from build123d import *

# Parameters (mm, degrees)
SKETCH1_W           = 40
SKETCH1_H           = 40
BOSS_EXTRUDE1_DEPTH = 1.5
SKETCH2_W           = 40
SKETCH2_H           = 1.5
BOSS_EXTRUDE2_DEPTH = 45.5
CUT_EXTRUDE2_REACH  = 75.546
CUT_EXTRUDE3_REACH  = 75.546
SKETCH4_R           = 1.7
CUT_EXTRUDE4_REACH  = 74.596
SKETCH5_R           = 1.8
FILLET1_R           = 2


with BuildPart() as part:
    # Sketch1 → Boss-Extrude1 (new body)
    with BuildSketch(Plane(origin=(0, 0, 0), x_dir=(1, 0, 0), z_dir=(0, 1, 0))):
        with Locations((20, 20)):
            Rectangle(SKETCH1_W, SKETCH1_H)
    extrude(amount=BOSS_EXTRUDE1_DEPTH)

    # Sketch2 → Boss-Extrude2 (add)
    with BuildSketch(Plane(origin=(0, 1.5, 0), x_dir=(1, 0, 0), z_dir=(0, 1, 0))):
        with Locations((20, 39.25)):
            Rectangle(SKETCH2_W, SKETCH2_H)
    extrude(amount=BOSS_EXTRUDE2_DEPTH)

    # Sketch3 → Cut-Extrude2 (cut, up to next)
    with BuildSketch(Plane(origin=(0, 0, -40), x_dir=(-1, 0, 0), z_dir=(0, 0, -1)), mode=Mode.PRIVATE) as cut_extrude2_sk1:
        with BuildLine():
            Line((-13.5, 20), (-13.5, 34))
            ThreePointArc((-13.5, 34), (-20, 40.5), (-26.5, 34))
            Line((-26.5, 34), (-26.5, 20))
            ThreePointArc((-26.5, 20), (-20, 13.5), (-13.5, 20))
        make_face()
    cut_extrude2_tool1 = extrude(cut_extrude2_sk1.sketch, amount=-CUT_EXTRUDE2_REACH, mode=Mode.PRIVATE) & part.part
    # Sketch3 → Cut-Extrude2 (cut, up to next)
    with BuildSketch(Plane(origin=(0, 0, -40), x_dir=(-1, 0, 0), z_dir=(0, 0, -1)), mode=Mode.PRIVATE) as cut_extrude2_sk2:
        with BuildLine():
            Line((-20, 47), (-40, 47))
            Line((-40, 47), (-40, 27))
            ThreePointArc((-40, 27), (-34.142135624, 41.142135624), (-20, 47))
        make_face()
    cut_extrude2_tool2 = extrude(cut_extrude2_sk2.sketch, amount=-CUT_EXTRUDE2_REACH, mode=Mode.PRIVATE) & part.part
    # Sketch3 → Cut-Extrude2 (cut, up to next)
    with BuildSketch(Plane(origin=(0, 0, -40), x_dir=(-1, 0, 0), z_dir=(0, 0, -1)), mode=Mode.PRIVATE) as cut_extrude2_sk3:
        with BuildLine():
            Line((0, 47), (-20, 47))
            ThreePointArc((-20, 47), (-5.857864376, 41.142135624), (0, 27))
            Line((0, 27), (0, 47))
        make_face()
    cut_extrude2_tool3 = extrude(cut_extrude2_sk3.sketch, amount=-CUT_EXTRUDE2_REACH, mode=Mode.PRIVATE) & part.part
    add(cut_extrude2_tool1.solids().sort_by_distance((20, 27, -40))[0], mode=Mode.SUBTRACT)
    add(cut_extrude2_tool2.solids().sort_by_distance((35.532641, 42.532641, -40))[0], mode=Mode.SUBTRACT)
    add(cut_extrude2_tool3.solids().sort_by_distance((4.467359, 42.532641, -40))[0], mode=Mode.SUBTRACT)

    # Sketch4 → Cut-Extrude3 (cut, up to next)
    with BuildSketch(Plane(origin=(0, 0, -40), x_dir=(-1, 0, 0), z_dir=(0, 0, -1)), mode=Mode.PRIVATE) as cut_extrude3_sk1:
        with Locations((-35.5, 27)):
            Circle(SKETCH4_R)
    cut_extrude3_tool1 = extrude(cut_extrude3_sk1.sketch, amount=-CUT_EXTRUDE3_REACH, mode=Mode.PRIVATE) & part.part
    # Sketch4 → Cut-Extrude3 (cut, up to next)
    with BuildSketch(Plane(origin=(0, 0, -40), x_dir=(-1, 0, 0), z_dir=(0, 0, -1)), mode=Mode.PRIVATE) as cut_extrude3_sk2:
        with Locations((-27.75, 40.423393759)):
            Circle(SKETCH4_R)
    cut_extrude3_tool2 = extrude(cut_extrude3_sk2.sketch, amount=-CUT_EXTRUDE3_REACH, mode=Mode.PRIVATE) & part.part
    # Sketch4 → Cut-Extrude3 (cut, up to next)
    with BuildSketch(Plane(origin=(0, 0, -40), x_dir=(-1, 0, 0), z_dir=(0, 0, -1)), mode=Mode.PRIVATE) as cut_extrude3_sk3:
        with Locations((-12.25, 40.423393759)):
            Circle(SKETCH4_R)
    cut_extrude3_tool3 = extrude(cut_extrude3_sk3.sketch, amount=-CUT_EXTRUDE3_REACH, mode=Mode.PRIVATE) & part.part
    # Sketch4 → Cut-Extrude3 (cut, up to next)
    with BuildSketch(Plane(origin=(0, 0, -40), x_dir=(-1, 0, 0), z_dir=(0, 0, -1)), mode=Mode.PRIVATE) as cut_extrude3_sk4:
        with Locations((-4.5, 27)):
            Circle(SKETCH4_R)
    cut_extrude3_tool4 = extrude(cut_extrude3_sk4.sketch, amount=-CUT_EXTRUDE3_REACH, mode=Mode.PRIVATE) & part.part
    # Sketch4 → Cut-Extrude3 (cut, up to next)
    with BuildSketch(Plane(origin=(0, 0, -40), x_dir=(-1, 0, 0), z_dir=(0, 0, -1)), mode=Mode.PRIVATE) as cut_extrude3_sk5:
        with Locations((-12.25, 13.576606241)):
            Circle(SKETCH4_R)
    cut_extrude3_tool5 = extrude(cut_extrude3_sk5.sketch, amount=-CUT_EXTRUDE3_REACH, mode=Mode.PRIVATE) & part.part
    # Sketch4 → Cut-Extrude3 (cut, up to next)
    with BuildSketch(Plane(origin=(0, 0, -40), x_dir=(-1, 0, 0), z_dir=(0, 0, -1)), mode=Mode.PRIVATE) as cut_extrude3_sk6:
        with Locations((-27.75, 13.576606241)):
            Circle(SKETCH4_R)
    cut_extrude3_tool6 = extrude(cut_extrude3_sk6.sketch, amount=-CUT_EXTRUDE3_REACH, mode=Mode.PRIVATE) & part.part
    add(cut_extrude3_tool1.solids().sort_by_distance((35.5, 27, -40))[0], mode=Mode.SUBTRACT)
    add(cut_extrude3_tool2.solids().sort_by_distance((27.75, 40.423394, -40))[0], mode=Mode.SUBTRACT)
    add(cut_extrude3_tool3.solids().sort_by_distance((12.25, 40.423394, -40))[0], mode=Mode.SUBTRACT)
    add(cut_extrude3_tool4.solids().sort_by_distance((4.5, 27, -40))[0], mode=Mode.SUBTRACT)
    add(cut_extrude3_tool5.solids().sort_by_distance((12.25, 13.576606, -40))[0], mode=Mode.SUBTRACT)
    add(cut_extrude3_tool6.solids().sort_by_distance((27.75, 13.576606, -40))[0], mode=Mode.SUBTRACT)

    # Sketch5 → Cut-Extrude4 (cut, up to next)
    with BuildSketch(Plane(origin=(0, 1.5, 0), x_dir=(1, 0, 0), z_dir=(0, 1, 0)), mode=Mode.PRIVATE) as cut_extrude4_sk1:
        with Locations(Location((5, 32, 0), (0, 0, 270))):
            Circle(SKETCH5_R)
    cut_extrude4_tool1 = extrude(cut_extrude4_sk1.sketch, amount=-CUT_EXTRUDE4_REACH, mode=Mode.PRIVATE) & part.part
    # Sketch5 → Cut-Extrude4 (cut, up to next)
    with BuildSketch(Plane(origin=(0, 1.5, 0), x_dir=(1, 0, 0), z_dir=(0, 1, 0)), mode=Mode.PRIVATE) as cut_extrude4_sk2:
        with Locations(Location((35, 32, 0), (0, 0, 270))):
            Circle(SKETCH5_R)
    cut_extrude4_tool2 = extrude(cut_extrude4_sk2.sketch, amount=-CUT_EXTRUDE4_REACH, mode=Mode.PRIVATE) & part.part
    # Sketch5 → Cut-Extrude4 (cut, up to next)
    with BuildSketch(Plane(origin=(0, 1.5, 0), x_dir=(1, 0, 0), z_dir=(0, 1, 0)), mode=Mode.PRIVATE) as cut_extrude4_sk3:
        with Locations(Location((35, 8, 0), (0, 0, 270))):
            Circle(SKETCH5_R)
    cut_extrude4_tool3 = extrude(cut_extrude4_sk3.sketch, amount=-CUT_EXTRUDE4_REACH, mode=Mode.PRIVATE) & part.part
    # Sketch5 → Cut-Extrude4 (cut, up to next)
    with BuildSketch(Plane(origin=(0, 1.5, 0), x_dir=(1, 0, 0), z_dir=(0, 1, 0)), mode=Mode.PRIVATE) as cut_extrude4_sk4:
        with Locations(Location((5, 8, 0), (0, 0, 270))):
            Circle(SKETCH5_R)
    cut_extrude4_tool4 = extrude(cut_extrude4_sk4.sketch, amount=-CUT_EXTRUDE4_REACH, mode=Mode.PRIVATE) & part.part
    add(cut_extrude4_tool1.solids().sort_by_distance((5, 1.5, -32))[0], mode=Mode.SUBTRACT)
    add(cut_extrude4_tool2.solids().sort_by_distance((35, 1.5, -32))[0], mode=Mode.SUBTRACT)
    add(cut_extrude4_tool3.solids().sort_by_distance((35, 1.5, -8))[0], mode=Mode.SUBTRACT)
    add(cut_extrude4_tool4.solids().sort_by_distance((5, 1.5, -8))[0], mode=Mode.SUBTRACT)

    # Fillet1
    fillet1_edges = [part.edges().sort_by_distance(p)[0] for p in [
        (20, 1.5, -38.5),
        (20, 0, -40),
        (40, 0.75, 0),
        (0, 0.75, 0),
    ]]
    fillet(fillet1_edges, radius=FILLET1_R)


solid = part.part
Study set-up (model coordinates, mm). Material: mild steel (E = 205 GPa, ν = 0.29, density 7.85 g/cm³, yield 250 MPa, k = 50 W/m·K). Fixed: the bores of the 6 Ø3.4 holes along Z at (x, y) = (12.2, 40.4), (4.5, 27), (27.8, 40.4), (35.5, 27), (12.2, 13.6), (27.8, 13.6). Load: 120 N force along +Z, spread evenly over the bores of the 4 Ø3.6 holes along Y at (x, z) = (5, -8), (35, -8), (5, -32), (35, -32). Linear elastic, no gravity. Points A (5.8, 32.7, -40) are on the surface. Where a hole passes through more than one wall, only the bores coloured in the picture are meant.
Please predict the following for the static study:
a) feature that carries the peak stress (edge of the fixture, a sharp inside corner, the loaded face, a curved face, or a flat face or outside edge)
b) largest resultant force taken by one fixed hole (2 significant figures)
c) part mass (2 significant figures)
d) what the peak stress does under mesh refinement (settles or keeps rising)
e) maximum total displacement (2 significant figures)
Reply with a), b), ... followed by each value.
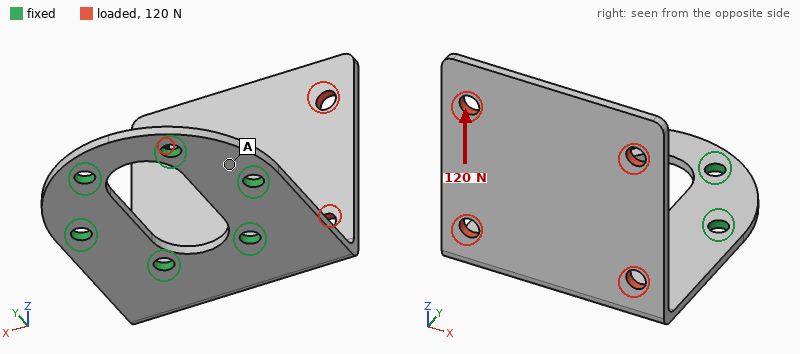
a) edge of the fixture
b) 71 N
c) 33 g
d) keeps rising
e) 0.16 mm
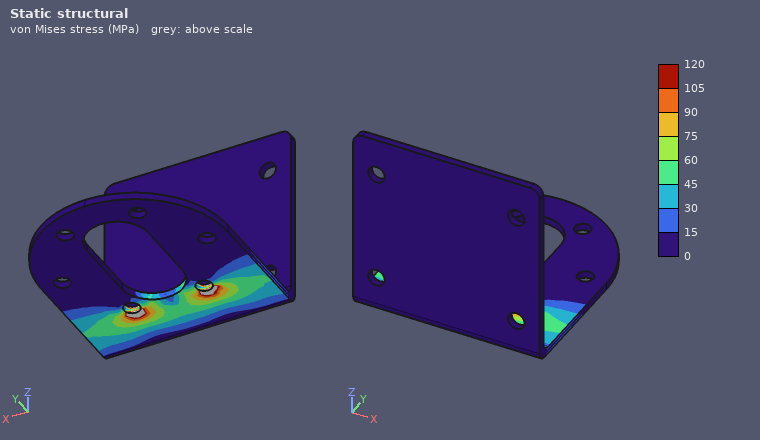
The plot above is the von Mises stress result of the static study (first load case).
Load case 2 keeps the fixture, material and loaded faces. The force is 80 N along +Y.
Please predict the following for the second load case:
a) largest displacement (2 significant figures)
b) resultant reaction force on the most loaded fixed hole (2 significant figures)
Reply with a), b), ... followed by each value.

a) 0.52 mm
b) 36 N
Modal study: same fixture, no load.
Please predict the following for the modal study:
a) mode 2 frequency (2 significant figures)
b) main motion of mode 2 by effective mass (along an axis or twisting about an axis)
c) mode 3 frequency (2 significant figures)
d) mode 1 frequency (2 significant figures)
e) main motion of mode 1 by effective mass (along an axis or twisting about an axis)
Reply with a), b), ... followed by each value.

a) 1300 Hz
b) along X
c) 2000 Hz
d) 560 Hz
e) along Y
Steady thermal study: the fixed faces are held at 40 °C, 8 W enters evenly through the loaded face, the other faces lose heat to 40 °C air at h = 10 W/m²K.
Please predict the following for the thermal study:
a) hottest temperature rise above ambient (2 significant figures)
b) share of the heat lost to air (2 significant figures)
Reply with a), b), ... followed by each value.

a) 75 K
b) 24 %
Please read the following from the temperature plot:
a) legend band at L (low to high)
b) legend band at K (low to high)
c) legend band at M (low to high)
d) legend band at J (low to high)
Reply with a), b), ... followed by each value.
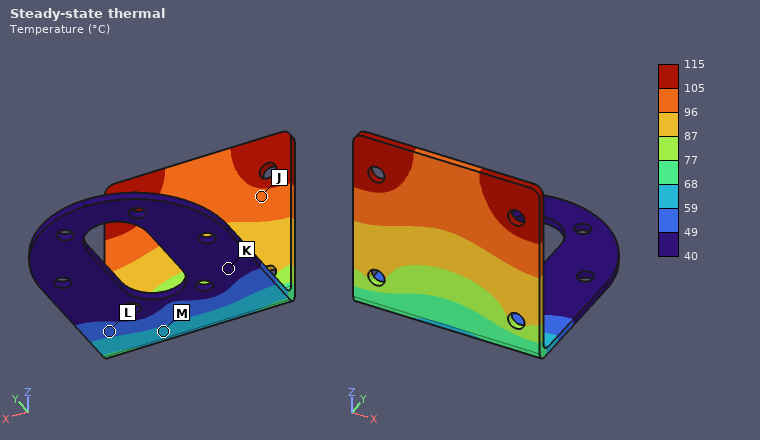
a) 49 to 59 °C
b) 40 to 49 °C
c) 59 to 68 °C
d) 96 to 105 °C
